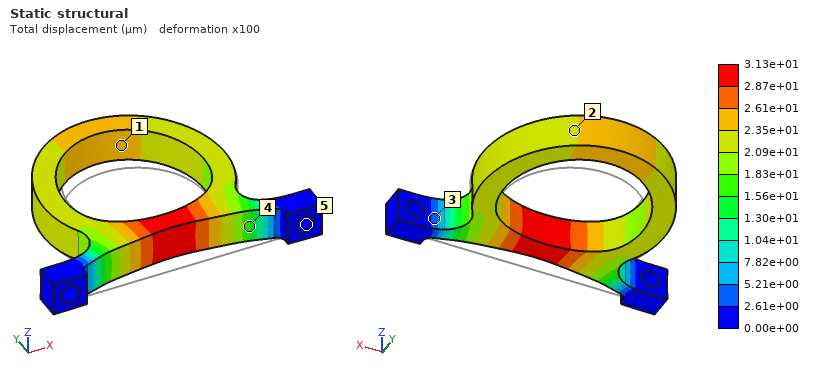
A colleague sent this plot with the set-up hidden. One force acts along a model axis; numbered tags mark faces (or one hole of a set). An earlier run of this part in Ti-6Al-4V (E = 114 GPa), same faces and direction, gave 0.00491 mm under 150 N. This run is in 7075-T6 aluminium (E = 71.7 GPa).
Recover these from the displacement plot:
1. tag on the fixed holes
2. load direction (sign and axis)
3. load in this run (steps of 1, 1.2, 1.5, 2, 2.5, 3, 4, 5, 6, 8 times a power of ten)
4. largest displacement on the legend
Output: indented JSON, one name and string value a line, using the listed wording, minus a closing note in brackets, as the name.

{
  "tag on the fixed holes": "5",
  "load direction": "+Y",
  "load in this run": "600 N",
  "largest displacement on the legend": "3.13e+01 µm"
}
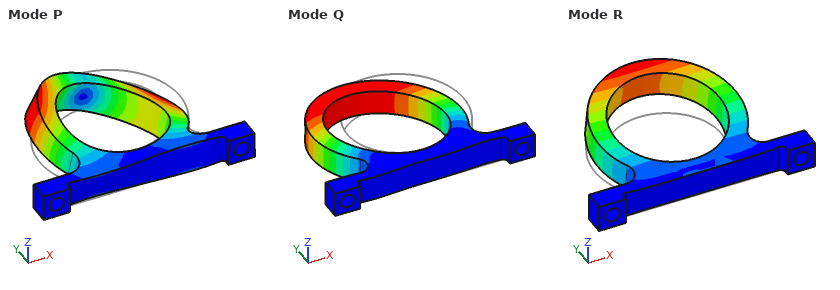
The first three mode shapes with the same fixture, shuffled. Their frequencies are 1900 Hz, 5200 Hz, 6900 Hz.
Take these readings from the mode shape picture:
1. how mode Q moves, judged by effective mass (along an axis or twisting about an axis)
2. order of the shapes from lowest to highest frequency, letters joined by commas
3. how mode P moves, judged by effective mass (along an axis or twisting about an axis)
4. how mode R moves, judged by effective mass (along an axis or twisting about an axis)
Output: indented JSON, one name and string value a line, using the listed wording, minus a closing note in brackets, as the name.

{
  "how mode Q moves, judged by effective mass": "along X",
  "order of the shapes from lowest to highest frequency, letters joined by commas": "R, Q, P",
  "how mode P moves, judged by effective mass": "twisting about Y",
  "how mode R moves, judged by effective mass": "along Z"
}
